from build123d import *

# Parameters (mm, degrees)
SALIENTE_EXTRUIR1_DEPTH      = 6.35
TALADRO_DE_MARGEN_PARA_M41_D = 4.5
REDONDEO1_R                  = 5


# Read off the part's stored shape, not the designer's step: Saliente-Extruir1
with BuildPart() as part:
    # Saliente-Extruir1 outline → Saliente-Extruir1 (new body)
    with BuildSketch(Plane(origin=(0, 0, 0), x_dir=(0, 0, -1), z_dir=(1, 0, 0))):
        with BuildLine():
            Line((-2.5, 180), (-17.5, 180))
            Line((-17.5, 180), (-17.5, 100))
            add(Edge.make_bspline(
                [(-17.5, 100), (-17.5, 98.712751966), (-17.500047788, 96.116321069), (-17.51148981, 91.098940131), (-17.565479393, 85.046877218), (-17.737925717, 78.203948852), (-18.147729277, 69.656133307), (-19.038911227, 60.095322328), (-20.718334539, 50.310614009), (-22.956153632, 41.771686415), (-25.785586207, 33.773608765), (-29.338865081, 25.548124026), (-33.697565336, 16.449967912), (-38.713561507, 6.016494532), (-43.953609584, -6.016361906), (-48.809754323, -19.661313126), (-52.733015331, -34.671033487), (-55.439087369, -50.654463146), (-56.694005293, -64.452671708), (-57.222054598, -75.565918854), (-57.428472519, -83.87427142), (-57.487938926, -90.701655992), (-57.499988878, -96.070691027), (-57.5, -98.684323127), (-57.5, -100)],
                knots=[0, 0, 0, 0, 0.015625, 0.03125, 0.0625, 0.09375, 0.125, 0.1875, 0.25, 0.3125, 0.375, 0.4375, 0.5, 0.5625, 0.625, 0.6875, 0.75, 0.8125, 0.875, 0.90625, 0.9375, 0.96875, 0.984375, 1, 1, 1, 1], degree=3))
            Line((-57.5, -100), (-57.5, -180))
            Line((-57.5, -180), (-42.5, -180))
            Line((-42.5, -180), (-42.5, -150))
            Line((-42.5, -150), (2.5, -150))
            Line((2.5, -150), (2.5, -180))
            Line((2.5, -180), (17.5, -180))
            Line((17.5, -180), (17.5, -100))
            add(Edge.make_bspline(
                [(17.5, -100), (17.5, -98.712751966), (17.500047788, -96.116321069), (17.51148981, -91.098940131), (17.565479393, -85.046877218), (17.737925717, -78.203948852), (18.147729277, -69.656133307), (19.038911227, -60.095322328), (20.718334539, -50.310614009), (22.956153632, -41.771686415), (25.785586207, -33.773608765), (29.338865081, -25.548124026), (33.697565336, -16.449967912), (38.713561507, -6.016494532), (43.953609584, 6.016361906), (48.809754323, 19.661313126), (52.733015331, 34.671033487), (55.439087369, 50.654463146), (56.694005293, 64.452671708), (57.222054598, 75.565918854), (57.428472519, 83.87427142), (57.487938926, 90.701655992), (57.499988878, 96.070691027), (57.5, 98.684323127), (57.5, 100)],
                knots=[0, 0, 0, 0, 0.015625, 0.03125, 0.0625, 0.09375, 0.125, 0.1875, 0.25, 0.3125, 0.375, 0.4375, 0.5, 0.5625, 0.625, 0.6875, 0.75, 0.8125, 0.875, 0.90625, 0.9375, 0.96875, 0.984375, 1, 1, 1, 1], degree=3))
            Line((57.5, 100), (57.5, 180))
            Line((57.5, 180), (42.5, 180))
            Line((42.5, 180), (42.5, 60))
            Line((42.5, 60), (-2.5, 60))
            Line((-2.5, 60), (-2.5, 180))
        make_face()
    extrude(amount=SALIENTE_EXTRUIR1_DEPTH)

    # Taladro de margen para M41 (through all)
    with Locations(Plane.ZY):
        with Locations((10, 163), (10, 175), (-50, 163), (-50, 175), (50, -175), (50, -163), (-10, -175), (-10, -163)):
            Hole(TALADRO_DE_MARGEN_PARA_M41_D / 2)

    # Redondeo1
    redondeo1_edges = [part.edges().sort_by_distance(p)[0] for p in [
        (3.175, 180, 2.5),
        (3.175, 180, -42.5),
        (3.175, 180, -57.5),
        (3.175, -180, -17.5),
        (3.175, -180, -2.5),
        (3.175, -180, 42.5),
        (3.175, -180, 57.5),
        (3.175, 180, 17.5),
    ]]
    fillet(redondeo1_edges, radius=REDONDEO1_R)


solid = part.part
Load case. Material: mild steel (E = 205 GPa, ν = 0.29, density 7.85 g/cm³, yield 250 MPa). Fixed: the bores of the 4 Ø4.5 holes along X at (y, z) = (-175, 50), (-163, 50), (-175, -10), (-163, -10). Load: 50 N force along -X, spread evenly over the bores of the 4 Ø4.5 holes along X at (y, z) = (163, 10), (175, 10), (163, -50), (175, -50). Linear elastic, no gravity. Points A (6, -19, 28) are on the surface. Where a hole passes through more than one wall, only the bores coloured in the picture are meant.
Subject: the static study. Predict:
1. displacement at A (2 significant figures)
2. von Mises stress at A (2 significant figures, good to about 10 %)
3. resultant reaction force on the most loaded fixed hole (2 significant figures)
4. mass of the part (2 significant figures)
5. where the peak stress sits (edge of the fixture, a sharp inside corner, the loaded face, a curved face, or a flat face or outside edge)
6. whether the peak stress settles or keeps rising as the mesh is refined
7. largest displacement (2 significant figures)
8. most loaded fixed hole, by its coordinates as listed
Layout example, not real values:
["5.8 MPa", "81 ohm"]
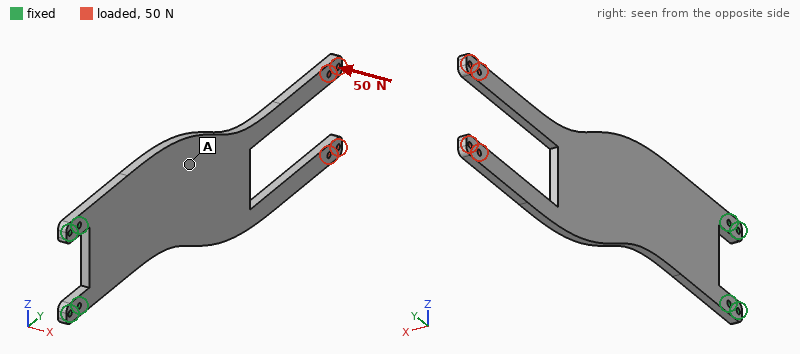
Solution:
["0.64 mm", "19 MPa", "200 N", "1.0 kg", "edge of the fixture", "keeps rising", "2.7 mm", "(-163, -10)"]
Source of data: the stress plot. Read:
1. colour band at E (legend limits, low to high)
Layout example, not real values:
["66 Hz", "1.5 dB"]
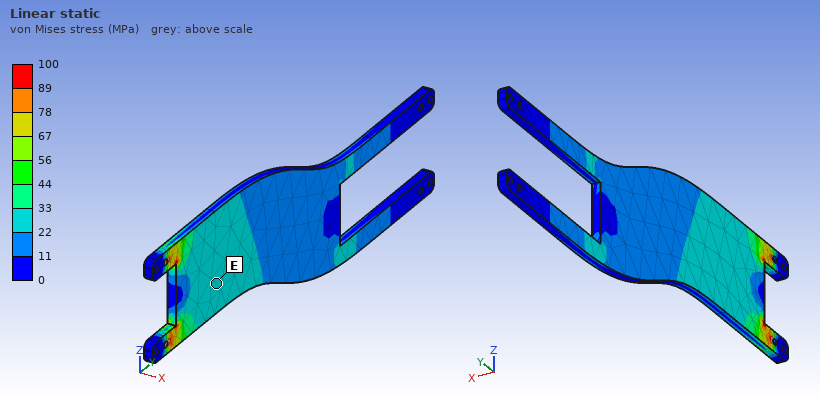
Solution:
["22 to 33 MPa"]
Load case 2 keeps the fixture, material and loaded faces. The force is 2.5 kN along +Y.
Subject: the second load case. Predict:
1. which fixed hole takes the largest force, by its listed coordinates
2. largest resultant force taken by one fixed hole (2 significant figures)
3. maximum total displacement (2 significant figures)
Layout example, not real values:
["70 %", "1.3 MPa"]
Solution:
["(-163, -10)", "2.5 kN", "0.13 mm"]
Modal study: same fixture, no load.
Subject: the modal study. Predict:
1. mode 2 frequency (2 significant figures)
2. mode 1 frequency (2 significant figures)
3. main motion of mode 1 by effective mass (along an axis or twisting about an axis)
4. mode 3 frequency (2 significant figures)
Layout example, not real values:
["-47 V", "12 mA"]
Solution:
["250 Hz", "53 Hz", "along X", "280 Hz"]
